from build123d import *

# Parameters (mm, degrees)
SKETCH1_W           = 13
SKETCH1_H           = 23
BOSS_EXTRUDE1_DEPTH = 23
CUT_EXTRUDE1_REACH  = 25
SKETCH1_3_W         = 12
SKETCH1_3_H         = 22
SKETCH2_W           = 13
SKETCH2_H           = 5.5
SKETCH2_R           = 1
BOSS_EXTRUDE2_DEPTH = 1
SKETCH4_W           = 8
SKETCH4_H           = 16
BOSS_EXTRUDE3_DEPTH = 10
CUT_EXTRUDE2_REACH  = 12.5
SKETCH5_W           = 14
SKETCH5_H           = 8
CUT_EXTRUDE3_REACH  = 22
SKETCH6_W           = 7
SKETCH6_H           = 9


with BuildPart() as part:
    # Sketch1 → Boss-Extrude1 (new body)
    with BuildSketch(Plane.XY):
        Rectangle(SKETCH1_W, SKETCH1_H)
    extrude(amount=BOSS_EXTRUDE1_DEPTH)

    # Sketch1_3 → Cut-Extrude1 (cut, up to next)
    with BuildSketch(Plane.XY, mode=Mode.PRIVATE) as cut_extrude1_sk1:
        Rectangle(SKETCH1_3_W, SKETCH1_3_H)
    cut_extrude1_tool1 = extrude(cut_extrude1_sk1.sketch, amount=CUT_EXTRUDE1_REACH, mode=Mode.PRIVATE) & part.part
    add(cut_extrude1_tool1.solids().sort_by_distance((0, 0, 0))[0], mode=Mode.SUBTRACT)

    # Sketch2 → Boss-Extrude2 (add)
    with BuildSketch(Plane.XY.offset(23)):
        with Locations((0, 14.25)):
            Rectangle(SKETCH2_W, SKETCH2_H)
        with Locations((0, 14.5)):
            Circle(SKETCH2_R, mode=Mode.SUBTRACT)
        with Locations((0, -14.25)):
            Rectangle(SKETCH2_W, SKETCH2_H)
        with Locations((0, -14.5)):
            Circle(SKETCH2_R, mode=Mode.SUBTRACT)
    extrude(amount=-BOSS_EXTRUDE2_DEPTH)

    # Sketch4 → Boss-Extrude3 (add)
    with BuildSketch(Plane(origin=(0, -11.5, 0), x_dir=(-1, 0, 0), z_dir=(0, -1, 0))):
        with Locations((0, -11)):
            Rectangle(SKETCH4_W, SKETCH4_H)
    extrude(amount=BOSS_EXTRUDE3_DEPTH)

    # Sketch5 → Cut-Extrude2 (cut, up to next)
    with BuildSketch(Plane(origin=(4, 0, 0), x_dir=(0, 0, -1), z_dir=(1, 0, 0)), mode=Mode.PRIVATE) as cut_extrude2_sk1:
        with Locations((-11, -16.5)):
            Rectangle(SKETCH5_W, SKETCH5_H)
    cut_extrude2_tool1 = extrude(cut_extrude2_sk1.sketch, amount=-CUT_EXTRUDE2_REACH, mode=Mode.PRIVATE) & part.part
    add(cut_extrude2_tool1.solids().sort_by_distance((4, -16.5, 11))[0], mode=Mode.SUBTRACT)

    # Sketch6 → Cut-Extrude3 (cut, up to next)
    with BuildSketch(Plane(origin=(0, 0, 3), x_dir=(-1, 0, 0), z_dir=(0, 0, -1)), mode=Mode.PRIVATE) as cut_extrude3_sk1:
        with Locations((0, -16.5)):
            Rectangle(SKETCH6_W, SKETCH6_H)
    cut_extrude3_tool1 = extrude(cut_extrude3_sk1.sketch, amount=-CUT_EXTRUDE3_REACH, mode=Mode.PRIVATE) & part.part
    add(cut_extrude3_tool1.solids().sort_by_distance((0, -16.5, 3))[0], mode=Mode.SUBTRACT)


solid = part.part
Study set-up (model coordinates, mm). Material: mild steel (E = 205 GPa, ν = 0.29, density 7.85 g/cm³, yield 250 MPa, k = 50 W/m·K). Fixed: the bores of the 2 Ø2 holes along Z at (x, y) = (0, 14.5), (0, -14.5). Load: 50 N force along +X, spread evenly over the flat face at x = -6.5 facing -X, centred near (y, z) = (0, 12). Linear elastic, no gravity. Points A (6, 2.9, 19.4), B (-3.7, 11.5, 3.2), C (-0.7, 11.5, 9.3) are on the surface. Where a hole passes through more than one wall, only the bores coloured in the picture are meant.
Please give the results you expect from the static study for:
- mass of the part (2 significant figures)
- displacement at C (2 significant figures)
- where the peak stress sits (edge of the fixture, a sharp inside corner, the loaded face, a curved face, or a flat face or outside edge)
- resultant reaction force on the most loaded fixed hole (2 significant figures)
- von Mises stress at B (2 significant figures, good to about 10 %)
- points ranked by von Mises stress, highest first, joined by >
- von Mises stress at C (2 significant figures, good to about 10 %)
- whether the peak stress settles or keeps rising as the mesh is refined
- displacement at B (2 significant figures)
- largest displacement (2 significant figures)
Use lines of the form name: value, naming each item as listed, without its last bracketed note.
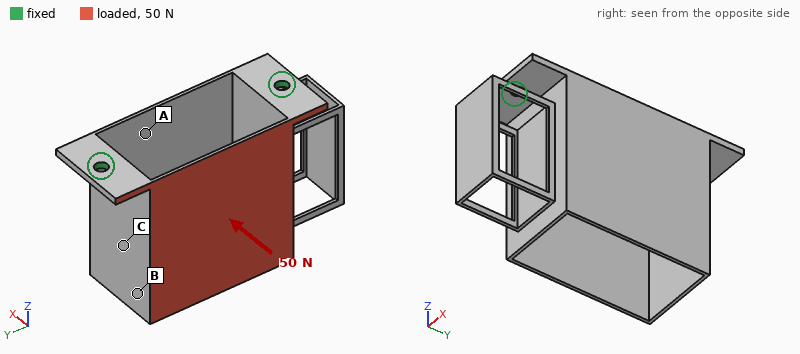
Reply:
mass of the part: 8.6 g
displacement at C: 0.033 mm
where the peak stress sits: edge of the fixture
resultant reaction force on the most loaded fixed hole: 26 N
von Mises stress at B: 42 MPa
points ranked by von Mises stress, highest first, joined by >: B > C > A
von Mises stress at C: 23 MPa
whether the peak stress settles or keeps rising as the mesh is refined: keeps rising
displacement at B: 0.047 mm
largest displacement: 0.11 mm
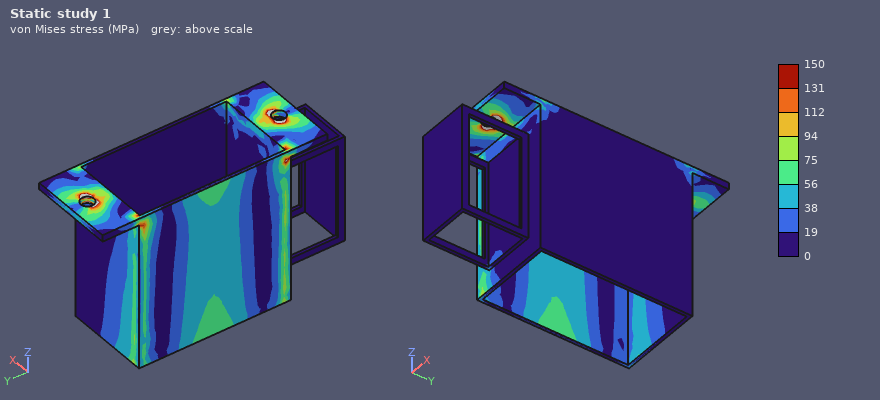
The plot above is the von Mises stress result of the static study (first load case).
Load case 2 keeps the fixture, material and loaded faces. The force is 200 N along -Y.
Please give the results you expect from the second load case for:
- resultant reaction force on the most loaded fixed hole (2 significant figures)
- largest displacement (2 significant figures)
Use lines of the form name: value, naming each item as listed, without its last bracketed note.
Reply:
resultant reaction force on the most loaded fixed hole: 130 N
largest displacement: 58 µm
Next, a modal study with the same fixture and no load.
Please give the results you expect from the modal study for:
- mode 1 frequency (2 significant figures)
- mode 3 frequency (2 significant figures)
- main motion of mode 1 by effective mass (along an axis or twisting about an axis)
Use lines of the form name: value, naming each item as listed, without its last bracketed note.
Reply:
mode 1 frequency: 1800 Hz
mode 3 frequency: 3500 Hz
main motion of mode 1 by effective mass: along X
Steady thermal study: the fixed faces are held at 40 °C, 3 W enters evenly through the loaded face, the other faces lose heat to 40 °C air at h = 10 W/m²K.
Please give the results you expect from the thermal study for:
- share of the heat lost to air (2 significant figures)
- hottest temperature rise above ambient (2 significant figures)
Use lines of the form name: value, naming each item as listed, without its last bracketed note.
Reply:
share of the heat lost to air: 24 %
hottest temperature rise above ambient: 45 K
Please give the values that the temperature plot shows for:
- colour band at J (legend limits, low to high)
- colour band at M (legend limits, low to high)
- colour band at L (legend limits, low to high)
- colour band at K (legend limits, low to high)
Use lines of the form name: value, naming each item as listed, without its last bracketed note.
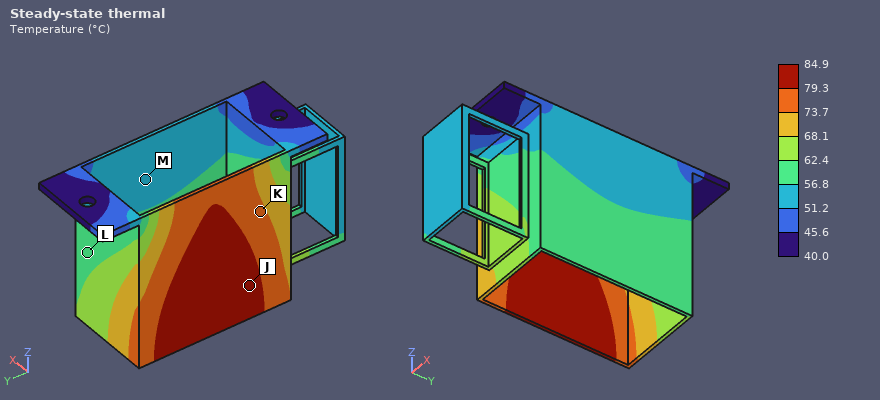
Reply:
colour band at J: 79.3 to 84.9 °C
colour band at M: 51.2 to 56.8 °C
colour band at L: 56.8 to 62.4 °C
colour band at K: 73.7 to 79.3 °C
